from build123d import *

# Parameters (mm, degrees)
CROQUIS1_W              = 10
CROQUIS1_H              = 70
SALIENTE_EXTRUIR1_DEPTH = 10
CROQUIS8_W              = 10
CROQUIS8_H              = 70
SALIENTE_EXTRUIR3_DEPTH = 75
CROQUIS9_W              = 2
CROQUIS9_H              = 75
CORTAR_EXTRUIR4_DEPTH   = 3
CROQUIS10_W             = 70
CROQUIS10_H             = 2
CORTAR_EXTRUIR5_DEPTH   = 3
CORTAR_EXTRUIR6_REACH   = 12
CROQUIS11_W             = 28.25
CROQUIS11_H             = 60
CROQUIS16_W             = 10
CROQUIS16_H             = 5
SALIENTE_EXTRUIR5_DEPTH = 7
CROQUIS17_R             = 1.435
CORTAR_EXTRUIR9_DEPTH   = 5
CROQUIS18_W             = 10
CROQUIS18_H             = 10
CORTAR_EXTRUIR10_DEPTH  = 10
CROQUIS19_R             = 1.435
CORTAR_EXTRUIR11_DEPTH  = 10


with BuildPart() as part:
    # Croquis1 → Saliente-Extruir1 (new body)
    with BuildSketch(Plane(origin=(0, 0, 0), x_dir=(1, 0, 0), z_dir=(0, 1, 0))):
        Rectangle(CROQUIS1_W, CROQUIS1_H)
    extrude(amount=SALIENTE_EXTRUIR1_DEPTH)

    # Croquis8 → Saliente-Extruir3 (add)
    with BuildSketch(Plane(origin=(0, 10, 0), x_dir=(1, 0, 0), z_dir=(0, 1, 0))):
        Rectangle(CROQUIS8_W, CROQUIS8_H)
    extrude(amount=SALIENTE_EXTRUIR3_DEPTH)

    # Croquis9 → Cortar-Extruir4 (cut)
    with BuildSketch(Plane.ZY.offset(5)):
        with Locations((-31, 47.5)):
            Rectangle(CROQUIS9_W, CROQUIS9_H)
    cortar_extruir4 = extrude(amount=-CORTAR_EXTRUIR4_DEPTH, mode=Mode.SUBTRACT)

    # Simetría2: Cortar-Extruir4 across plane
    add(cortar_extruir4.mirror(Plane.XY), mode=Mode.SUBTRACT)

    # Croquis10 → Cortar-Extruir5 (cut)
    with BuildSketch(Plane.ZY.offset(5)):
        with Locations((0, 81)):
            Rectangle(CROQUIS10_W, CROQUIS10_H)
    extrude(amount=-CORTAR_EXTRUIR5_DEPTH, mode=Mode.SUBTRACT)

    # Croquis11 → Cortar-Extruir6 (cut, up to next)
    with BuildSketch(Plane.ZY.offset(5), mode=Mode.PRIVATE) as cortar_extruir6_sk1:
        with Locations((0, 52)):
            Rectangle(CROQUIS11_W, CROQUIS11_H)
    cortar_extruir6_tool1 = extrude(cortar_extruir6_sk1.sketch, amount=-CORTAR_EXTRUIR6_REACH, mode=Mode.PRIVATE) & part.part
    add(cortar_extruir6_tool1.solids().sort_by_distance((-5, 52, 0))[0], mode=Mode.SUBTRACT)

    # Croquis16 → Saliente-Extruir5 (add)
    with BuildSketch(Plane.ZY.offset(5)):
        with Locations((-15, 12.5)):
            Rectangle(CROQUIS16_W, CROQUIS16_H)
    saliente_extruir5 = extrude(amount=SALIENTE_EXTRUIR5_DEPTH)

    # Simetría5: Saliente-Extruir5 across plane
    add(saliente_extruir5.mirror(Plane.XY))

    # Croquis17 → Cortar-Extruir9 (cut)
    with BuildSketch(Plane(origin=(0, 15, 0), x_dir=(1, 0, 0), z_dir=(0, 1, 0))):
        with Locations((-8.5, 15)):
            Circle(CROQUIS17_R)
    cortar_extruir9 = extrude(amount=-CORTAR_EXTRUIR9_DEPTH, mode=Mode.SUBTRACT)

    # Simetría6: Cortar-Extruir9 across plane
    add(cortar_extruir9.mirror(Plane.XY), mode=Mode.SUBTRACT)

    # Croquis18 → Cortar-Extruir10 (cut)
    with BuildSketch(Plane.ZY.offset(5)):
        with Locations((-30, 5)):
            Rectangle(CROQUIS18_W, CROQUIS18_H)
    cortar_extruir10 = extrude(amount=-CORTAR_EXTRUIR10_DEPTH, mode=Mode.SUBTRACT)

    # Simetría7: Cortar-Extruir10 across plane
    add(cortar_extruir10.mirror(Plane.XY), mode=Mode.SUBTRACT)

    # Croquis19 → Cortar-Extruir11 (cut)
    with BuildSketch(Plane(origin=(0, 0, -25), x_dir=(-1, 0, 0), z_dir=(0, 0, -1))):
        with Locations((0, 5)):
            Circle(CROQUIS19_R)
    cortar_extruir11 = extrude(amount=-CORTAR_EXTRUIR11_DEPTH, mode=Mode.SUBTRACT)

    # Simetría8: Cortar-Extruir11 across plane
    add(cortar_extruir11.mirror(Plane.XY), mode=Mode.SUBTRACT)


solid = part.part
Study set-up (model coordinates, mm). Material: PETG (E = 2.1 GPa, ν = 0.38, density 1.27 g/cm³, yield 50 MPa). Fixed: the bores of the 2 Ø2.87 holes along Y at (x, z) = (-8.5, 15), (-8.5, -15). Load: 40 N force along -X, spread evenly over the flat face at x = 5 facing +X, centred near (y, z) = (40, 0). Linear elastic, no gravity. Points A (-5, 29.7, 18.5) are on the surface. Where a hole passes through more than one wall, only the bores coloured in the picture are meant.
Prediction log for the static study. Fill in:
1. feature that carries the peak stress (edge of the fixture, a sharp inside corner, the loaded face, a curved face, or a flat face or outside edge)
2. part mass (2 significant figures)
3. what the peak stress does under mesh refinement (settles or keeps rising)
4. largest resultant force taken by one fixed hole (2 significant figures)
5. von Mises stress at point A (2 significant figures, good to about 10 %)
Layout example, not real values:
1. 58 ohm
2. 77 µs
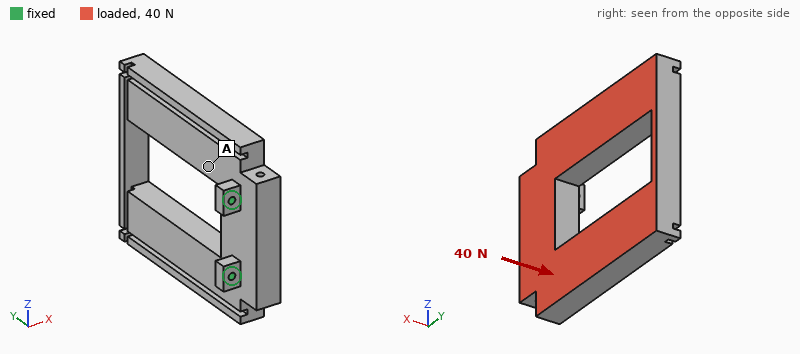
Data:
1. edge of the fixture
2. 51 g
3. keeps rising
4. 21 N
5. 1.1 MPa
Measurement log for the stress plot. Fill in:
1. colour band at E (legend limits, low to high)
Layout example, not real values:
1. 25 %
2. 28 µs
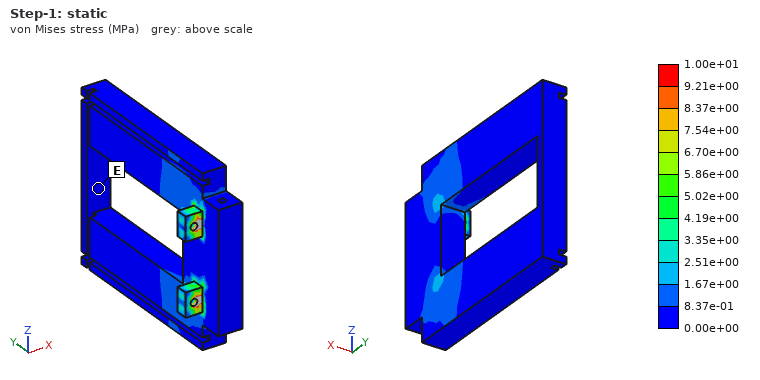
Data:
1. 0.00e+00 to 8.37e-01 MPa
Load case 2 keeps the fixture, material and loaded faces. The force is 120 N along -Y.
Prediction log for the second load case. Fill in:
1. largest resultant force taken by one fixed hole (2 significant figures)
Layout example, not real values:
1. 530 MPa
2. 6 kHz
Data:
1. 60 N
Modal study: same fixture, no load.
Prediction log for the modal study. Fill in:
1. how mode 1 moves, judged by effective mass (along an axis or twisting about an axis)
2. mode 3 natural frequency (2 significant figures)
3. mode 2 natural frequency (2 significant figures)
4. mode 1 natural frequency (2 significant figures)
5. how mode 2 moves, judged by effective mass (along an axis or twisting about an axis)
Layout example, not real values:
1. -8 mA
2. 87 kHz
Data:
1. along X
2. 530 Hz
3. 430 Hz
4. 160 Hz
5. along Z
